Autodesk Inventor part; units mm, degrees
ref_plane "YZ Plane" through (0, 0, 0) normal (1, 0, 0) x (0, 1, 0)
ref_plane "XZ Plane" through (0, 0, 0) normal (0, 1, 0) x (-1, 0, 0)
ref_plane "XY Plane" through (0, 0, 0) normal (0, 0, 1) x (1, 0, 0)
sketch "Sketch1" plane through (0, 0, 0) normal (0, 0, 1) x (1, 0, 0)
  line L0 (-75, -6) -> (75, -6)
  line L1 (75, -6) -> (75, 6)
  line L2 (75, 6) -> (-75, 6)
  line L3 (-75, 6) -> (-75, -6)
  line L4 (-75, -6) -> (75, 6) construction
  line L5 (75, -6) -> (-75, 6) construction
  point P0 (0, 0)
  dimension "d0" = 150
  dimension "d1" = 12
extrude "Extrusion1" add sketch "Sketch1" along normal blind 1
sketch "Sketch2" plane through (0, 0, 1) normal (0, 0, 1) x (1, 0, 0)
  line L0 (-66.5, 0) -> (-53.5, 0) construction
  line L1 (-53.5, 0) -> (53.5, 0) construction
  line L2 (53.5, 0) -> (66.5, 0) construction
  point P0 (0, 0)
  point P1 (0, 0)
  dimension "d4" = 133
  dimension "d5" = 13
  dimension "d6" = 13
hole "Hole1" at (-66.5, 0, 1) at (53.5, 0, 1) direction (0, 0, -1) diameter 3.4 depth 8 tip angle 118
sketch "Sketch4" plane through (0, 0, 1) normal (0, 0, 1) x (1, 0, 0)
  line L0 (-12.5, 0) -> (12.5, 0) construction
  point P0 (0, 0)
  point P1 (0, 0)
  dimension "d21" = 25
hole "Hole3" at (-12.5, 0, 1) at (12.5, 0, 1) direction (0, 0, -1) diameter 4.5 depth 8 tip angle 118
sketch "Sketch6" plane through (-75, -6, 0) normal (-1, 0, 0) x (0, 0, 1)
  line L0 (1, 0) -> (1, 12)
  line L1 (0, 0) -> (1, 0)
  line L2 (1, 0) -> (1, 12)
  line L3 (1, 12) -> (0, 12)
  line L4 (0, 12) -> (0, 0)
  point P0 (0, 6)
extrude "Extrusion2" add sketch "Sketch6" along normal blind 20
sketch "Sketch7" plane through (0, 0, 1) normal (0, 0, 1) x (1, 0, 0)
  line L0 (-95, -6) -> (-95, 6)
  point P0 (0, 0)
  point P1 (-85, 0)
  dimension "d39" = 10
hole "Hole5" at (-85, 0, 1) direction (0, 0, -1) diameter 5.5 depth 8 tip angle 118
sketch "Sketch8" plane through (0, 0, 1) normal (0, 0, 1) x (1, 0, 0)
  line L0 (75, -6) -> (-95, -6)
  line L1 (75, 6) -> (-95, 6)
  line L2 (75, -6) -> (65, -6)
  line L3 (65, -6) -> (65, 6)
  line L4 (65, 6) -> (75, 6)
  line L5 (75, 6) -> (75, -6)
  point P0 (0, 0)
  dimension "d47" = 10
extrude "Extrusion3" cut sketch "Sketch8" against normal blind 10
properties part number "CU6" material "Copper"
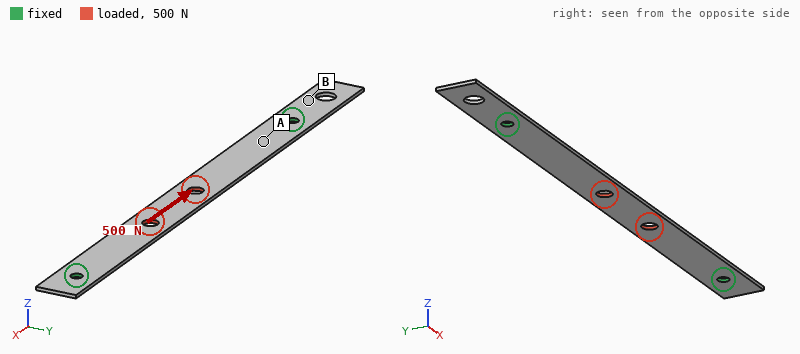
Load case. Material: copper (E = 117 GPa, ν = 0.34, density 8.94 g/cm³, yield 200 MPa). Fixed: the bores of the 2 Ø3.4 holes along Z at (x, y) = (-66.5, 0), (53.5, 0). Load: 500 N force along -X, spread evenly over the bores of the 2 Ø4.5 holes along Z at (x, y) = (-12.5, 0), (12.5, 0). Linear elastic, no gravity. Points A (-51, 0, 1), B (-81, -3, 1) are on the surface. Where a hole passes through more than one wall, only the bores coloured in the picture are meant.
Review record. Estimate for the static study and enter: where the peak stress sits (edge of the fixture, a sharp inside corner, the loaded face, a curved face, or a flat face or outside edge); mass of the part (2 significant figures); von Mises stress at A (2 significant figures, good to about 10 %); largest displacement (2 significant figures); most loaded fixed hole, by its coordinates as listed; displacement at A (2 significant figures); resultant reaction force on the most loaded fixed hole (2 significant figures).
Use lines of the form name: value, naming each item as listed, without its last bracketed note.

where the peak stress sits: the loaded face
mass of the part: 17 g
von Mises stress at A: 19 MPa
largest displacement: 9.7 µm
most loaded fixed hole, by its coordinates as listed: (53.5, 0)
displacement at A: 2.8 µm
resultant reaction force on the most loaded fixed hole: 270 N
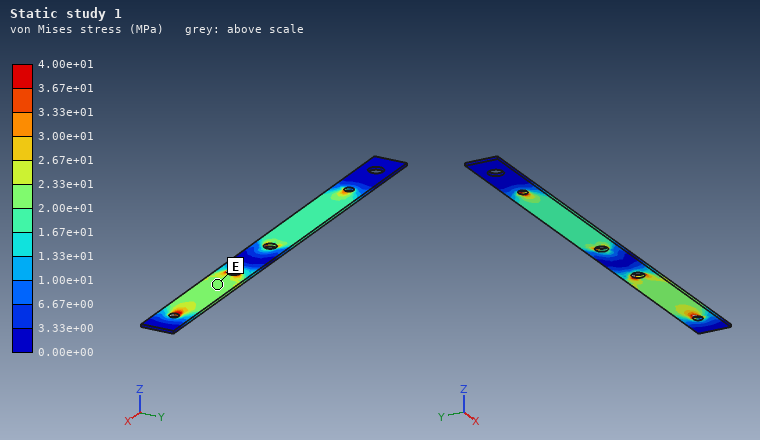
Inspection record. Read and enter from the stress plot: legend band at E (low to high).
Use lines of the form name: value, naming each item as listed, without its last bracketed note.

legend band at E: 2.00e+01 to 2.33e+01 MPa
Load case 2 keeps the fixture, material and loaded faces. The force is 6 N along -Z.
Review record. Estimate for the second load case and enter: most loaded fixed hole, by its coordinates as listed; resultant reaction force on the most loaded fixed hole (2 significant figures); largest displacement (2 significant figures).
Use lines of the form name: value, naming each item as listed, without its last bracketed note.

most loaded fixed hole, by its coordinates as listed: (53.5, 0)
resultant reaction force on the most loaded fixed hole: 3.5 N
largest displacement: 0.39 mm
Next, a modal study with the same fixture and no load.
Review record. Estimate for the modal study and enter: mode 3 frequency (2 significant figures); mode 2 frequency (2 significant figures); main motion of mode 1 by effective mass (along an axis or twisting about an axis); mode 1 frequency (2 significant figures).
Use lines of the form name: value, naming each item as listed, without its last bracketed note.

mode 3 frequency: 810 Hz
mode 2 frequency: 740 Hz
main motion of mode 1 by effective mass: along Z
mode 1 frequency: 270 Hz
